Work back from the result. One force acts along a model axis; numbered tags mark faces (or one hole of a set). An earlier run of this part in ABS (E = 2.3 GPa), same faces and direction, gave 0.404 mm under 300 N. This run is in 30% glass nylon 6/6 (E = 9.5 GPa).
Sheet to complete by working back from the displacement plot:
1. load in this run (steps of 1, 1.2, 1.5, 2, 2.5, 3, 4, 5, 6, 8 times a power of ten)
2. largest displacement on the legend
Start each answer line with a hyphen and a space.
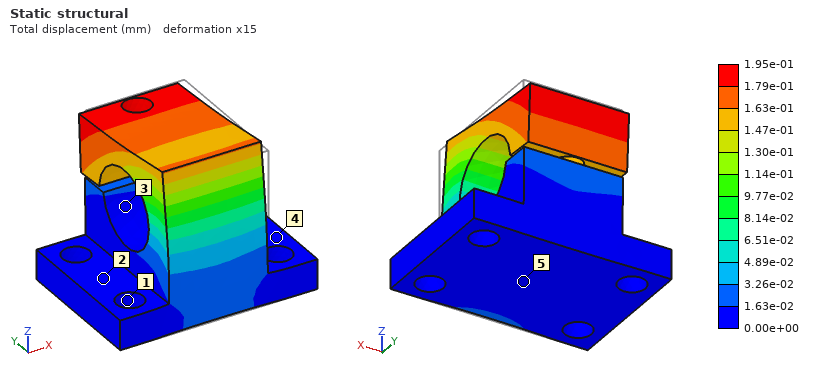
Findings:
- 600 N
- 1.95e-01 mm
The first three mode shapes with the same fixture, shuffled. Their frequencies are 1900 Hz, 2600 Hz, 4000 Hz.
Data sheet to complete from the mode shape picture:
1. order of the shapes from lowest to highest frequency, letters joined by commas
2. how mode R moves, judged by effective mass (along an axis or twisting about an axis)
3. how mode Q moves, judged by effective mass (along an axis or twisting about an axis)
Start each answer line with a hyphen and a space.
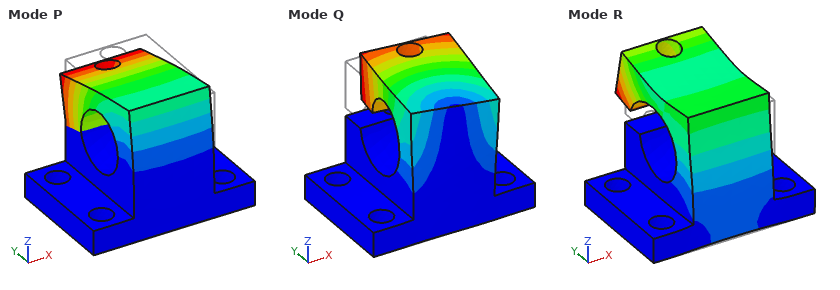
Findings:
- P, Q, R
- along Y
- along X
